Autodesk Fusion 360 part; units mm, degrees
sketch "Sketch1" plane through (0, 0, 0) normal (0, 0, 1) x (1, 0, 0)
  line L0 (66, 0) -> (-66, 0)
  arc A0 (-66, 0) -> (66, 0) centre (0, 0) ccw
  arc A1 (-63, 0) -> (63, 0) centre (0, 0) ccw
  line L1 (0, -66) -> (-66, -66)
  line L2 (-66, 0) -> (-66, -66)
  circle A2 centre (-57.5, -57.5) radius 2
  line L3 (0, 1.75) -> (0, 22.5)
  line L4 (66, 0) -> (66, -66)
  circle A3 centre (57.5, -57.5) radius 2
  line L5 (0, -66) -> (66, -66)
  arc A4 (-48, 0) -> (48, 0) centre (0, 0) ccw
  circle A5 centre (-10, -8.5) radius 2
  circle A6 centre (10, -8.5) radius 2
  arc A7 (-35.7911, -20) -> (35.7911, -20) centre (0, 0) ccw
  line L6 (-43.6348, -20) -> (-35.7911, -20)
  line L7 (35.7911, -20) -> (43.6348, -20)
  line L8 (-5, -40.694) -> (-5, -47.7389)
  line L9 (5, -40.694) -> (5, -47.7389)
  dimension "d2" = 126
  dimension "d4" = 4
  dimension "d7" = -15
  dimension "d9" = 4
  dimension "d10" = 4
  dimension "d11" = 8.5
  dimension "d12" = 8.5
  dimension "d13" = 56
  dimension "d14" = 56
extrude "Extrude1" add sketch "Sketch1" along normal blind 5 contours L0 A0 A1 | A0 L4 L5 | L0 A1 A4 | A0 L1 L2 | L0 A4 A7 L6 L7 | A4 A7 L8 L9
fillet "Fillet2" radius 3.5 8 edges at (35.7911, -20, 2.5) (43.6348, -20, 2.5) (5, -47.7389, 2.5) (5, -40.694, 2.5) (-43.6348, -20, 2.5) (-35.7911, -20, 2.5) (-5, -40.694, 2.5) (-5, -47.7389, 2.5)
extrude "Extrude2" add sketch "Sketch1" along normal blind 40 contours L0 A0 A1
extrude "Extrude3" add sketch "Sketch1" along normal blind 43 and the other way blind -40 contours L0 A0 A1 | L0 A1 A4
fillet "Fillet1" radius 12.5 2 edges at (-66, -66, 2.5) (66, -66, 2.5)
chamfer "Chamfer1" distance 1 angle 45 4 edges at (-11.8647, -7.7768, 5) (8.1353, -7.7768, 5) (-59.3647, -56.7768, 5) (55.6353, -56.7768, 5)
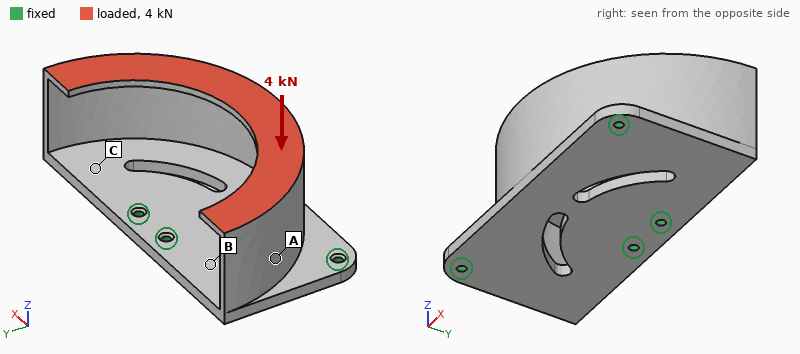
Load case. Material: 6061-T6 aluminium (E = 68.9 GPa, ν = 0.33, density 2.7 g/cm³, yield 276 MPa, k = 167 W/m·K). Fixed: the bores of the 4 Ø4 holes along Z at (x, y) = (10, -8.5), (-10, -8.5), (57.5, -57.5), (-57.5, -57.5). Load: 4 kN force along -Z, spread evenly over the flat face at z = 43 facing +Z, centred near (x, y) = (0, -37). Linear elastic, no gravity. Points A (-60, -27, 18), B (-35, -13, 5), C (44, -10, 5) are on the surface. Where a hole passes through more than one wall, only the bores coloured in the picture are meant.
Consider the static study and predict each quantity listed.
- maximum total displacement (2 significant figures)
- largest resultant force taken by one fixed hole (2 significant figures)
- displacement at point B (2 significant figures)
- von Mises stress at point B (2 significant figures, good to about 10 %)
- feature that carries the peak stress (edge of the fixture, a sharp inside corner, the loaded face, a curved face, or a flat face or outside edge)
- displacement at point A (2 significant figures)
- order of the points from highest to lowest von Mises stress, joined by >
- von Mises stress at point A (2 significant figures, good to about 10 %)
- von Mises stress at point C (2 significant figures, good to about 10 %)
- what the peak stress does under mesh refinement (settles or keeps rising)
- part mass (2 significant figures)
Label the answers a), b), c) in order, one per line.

a) 0.68 mm
b) 1.4 kN
c) 0.14 mm
d) 26 MPa
e) edge of the fixture
f) 0.25 mm
g) C > B > A
h) 14 MPa
i) 43 MPa
j) keeps rising
k) 190 g
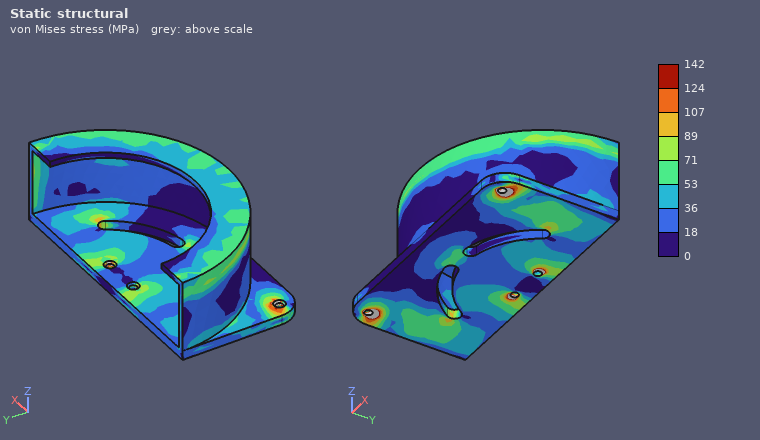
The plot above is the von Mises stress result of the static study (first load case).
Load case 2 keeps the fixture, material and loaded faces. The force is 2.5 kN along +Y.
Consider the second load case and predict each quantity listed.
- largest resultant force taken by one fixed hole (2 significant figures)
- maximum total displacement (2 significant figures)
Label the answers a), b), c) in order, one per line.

a) 1.2 kN
b) 1.1 mm
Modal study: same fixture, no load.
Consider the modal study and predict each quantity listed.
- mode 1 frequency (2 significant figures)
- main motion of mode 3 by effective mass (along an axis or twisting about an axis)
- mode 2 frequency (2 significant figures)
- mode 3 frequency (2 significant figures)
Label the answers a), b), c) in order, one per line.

a) 1100 Hz
b) along Z
c) 1400 Hz
d) 2400 Hz
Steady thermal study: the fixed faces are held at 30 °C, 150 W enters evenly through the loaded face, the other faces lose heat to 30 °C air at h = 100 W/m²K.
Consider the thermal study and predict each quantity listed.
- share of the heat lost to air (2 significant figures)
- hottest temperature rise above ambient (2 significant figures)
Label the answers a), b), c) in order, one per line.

a) 63 %
b) 63 K
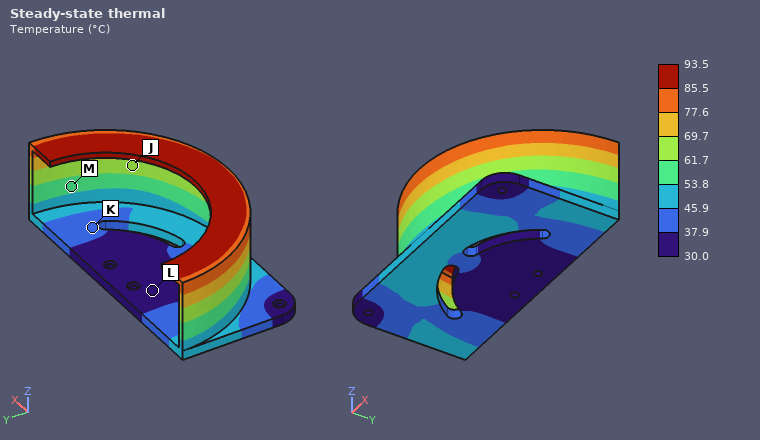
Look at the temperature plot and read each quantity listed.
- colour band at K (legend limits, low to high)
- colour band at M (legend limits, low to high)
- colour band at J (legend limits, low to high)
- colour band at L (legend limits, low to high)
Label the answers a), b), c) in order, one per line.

a) 37.9 to 45.9 °C
b) 53.8 to 61.7 °C
c) 61.7 to 69.7 °C
d) 30.0 to 37.9 °C
